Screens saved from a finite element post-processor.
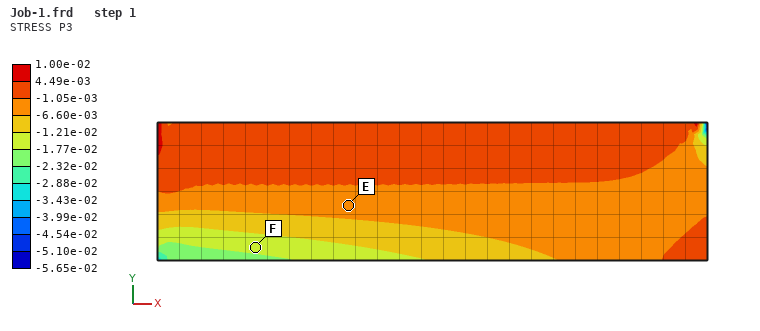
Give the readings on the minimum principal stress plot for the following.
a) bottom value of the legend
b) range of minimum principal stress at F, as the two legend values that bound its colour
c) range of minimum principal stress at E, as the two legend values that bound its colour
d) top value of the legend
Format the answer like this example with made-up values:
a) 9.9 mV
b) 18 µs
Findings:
a) -5.65e-02
b) -1.77e-02 to -1.21e-02
c) -6.60e-03 to -1.05e-03
d) 1.00e-02
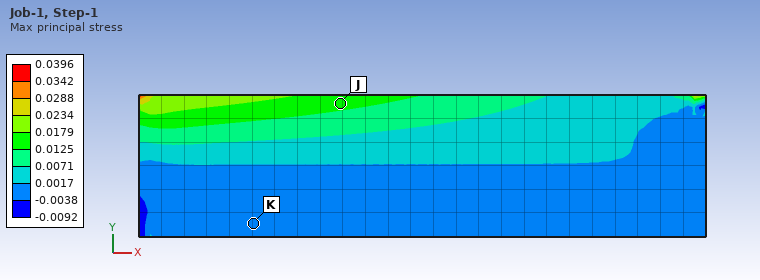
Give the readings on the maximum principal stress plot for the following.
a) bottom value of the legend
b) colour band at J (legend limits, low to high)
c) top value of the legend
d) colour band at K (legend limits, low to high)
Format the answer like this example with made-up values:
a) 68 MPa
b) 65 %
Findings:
a) -0.0092
b) 0.0125 to 0.0179
c) 0.0396
d) -0.0038 to 0.0017
